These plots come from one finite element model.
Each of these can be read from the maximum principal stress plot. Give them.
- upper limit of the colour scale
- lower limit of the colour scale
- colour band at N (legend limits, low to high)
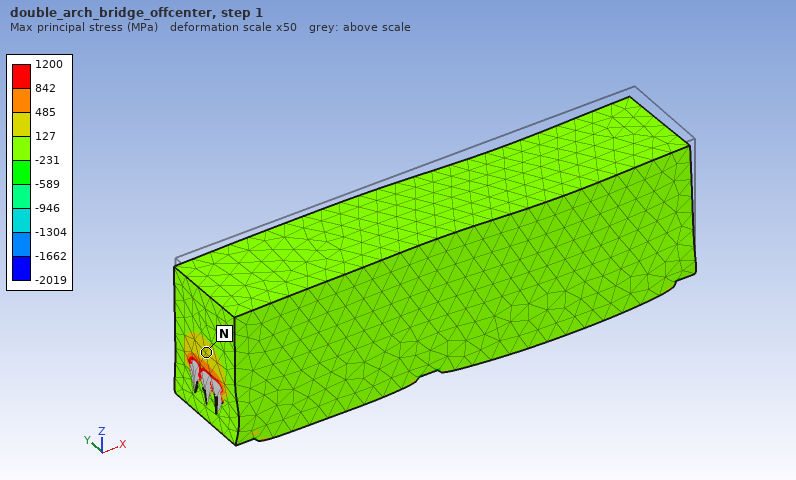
1200 MPa
-2019 MPa
127 to 485 MPa
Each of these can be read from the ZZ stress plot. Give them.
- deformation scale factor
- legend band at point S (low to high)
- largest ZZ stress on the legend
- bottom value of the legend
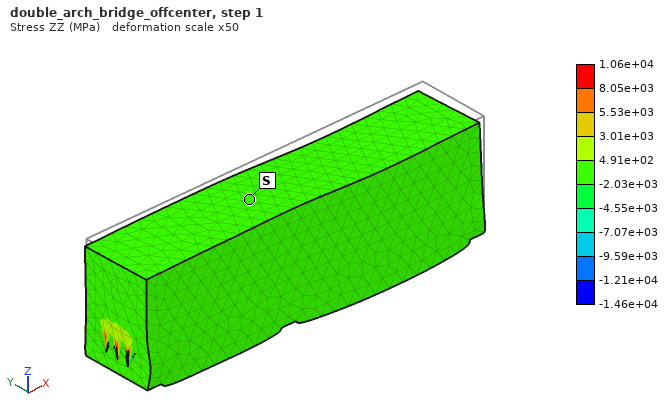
50
-2.03e+03 to 4.91e+02 MPa
1.06e+04 MPa
-1.46e+04 MPa
